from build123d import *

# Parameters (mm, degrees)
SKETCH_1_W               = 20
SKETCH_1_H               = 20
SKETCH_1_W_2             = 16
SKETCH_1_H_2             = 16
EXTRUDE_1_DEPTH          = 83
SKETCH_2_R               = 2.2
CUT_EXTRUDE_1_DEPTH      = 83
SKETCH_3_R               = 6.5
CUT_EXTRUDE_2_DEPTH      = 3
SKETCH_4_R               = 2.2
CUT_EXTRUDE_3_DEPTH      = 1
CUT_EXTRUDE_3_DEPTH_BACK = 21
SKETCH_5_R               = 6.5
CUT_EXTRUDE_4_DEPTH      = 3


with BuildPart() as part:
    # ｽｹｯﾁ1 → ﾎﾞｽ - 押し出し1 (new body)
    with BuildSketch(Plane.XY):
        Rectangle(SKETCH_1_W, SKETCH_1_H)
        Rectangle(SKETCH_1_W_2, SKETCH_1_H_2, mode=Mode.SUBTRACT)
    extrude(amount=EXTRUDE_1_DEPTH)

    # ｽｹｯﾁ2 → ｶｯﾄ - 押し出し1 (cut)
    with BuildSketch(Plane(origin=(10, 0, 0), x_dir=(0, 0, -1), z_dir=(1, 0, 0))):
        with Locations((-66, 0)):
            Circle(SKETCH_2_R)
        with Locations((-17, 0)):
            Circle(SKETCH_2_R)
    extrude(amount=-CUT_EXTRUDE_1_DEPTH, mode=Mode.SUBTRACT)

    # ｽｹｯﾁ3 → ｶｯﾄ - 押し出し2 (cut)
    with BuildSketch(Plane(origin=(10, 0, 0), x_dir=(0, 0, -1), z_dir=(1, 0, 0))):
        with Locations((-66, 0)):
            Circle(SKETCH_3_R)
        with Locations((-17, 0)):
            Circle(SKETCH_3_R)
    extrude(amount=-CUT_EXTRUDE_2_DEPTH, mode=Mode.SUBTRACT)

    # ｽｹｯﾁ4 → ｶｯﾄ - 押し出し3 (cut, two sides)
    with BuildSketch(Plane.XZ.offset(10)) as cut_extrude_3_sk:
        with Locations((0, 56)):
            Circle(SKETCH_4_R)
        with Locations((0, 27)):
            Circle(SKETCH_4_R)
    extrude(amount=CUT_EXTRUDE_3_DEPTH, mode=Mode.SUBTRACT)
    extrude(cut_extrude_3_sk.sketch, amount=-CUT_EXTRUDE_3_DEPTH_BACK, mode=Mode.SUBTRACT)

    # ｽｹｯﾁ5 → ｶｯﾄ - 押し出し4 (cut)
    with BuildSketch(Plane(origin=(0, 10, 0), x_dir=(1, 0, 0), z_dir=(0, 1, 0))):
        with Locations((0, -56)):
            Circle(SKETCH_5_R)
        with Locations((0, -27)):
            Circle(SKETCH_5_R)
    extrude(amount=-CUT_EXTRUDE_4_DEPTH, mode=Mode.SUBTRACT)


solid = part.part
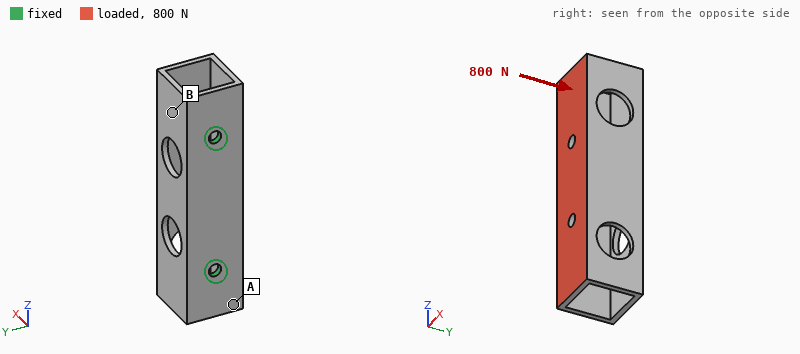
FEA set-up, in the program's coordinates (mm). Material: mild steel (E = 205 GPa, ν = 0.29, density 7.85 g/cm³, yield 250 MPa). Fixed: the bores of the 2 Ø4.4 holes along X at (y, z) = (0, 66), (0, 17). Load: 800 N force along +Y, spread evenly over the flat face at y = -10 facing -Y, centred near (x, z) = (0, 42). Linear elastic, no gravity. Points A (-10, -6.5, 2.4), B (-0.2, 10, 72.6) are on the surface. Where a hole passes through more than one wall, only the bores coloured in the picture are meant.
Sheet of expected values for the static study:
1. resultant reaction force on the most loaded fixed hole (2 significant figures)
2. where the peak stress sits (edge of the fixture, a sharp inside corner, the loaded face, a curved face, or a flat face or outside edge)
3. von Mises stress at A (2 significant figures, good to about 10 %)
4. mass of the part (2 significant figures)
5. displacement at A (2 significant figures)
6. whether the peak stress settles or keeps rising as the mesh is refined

400 N
edge of the fixture
38 MPa
85 g
13 µm
keeps rising
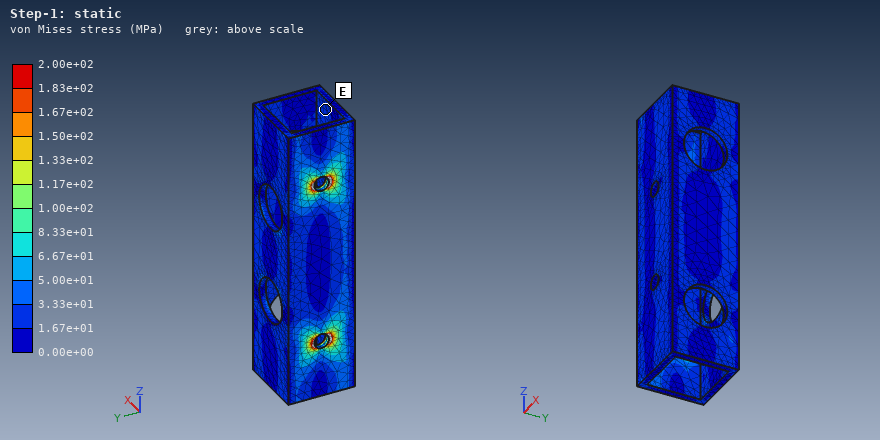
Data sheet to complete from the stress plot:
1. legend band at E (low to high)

1.67e+01 to 3.33e+01 MPa
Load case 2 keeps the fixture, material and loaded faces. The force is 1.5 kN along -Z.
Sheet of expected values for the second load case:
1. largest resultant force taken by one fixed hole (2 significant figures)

840 N
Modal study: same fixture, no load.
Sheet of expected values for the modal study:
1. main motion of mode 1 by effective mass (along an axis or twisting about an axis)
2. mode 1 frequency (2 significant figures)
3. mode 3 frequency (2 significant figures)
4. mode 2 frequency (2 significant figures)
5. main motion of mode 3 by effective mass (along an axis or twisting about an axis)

along Y
2100 Hz
5900 Hz
5400 Hz
along X
